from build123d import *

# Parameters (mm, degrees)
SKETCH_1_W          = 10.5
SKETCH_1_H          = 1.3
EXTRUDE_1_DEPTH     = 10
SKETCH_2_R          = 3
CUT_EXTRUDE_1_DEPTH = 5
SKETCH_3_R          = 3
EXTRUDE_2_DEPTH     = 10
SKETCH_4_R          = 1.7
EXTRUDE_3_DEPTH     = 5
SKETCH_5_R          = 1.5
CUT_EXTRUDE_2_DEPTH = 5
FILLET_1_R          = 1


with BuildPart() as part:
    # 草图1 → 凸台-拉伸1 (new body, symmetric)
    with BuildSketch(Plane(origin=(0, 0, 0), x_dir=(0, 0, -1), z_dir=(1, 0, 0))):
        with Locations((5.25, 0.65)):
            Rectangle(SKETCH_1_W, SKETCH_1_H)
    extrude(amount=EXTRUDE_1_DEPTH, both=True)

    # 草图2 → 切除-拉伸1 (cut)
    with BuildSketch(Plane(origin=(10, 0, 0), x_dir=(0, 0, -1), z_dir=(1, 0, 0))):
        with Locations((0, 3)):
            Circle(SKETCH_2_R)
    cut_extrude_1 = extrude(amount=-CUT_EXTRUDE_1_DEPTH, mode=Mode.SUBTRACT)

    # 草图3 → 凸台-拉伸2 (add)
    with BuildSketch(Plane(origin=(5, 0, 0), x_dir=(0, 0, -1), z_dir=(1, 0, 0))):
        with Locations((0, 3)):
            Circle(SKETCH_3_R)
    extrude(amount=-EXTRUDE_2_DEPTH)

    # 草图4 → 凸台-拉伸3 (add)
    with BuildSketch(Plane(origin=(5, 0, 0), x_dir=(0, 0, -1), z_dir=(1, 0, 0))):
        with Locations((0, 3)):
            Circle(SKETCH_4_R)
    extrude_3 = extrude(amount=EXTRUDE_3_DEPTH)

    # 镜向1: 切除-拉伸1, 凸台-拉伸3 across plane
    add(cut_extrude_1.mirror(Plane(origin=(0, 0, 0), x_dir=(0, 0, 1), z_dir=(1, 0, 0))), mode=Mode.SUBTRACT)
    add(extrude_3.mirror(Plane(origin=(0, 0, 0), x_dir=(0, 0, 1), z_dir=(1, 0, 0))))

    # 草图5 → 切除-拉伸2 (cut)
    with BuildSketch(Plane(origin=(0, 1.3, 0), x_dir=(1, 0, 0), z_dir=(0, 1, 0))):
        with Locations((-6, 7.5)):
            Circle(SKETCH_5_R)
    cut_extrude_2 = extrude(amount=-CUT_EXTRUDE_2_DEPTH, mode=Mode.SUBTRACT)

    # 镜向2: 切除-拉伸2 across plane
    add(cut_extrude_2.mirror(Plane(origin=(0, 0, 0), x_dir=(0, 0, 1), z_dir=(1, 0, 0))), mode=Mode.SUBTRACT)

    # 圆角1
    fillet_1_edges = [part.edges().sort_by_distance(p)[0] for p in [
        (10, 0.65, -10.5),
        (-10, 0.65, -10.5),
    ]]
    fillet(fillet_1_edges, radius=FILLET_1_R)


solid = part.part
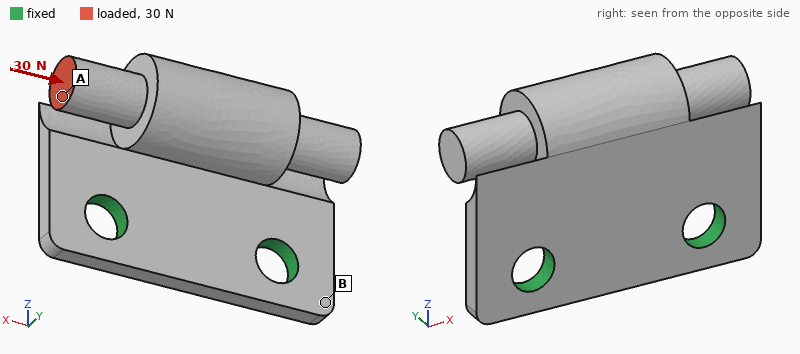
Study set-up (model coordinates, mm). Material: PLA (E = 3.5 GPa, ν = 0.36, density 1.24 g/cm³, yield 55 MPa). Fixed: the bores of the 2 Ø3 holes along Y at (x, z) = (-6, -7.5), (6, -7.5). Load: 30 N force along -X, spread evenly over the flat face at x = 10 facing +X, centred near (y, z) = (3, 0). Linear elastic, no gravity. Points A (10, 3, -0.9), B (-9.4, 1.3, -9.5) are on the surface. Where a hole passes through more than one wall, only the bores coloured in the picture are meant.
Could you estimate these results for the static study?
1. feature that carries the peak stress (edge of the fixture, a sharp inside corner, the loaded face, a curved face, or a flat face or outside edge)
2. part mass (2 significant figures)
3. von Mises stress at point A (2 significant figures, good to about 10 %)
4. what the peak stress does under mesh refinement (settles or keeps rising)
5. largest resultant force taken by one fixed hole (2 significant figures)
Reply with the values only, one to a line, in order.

a sharp inside corner
0.72 g
3.3 MPa
keeps rising
23 N
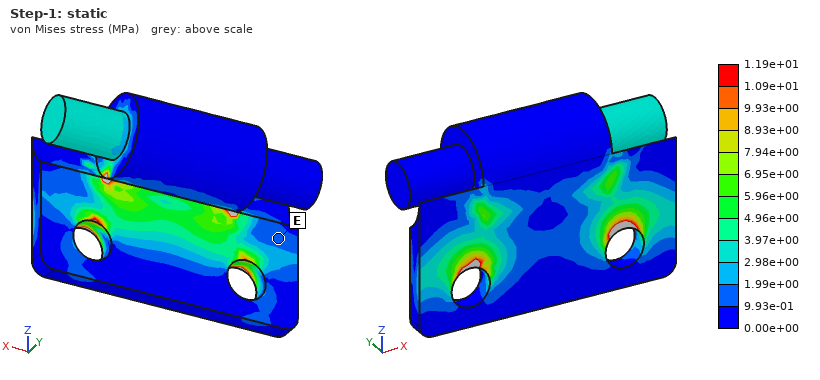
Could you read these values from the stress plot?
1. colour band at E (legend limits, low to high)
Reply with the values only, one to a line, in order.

9.93e-01 to 1.99e+00 MPa
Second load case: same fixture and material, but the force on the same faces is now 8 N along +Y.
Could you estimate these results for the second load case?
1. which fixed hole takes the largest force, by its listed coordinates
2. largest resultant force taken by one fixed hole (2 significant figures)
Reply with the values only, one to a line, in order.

(6, -7.5)
12 N
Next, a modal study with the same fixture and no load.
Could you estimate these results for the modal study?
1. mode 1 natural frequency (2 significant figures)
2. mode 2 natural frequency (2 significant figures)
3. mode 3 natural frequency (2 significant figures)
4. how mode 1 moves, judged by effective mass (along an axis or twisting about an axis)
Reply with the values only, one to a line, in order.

2000 Hz
4900 Hz
8900 Hz
along Y
